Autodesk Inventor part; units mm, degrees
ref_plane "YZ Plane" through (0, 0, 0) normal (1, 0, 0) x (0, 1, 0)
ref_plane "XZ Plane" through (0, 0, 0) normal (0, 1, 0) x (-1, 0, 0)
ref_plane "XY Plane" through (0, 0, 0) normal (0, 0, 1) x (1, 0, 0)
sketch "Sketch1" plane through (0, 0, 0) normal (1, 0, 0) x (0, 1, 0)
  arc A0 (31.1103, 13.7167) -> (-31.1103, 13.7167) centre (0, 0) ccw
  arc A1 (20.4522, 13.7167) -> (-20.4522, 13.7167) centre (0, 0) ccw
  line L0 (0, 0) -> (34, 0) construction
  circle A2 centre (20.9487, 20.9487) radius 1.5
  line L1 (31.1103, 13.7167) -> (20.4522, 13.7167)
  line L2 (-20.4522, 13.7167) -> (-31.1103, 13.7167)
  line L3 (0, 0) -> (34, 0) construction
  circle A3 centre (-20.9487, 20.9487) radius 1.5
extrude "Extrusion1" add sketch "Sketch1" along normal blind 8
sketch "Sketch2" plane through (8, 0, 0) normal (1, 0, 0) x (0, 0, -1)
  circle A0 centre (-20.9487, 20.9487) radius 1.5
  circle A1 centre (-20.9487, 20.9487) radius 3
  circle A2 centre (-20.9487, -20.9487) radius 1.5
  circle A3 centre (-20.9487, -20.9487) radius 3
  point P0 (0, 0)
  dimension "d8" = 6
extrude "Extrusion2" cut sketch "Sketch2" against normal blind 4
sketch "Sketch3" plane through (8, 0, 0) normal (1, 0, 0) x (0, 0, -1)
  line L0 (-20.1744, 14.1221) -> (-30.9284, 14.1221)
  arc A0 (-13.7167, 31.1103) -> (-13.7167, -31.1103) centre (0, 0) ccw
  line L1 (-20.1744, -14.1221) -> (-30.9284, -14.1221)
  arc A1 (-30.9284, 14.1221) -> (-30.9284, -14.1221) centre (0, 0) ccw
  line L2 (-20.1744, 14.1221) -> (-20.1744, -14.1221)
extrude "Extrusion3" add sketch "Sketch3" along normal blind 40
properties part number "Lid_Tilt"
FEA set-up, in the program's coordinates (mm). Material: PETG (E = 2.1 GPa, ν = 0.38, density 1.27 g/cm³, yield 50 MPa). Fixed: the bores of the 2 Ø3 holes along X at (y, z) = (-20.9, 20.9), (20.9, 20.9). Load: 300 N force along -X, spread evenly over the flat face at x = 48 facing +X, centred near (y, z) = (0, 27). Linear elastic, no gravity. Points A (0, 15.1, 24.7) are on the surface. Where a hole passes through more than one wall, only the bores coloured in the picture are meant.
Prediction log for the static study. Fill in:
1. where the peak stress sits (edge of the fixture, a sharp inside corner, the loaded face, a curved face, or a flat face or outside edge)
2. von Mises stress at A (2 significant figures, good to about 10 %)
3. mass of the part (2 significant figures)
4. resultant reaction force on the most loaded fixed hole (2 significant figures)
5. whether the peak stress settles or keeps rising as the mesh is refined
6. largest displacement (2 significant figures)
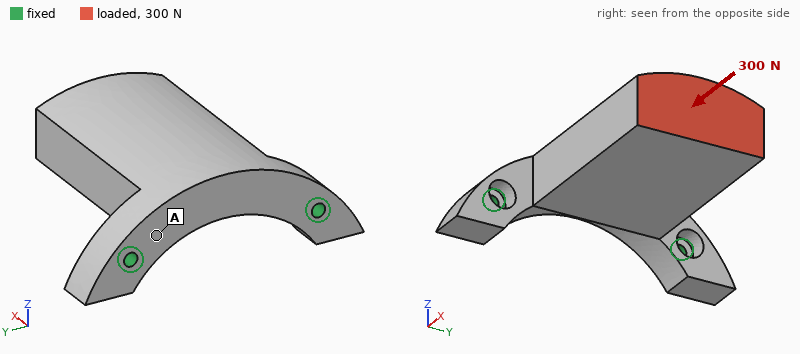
edge of the fixture
4.5 MPa
24 g
160 N
keeps rising
0.82 mm
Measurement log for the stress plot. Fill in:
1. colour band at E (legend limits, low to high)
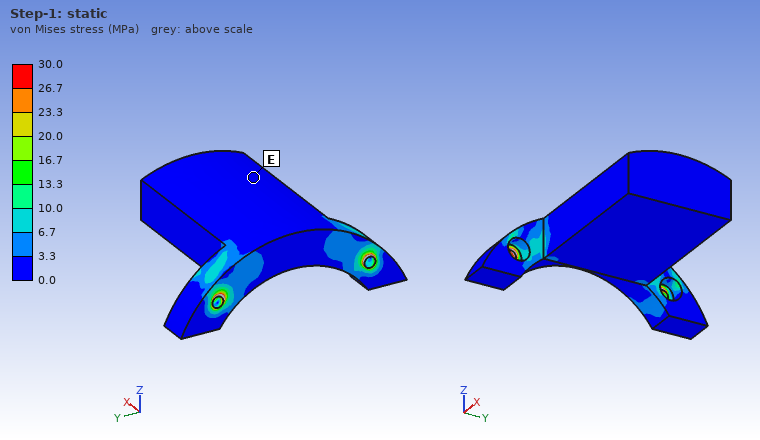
0.0 to 3.3 MPa
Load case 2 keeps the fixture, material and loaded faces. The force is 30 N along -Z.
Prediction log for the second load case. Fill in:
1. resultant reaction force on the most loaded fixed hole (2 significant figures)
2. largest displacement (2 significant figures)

20 N
0.93 mm
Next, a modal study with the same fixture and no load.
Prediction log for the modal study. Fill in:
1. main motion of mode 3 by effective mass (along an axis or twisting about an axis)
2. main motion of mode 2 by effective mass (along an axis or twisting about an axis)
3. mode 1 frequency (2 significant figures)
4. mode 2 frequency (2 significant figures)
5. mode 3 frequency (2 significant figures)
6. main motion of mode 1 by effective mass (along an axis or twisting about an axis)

along X
along Y
350 Hz
1400 Hz
2100 Hz
along Z
